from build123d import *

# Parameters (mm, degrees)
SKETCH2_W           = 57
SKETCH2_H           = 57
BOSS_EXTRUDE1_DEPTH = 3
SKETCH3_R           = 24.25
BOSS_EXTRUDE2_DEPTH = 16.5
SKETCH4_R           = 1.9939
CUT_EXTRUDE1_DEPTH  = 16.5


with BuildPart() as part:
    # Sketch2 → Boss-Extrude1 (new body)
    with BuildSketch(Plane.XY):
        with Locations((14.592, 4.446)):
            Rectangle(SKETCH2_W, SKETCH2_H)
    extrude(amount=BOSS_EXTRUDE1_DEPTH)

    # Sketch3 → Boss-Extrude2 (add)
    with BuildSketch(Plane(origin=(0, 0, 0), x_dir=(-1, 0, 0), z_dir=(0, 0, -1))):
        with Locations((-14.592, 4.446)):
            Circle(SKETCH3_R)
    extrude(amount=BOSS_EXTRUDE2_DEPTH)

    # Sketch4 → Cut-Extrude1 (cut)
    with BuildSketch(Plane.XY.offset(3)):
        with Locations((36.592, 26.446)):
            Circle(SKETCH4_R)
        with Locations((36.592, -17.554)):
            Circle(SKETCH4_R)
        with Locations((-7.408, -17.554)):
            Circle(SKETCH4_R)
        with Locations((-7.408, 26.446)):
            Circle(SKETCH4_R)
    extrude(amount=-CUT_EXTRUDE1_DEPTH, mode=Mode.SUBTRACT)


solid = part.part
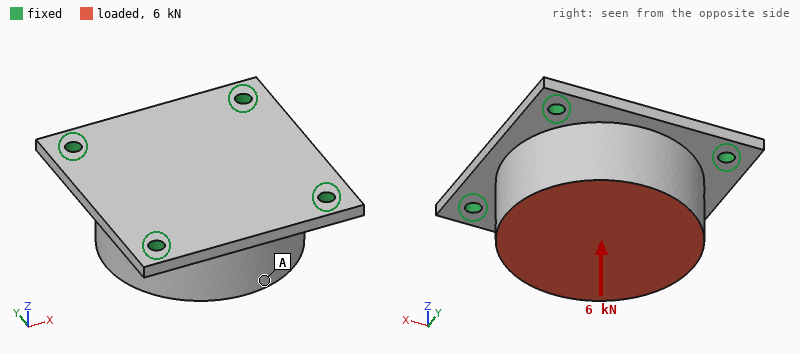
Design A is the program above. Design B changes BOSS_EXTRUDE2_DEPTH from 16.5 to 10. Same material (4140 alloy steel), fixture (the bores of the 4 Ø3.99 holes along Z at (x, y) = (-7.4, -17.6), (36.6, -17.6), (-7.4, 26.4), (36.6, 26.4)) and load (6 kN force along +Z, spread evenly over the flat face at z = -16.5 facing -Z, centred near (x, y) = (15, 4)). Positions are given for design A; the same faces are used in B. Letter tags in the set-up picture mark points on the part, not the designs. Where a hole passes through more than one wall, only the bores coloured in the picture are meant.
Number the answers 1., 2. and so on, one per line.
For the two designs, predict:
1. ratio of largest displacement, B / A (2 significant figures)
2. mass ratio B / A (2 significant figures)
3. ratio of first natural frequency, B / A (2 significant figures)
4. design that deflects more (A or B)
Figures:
1. 1.1
2. 0.70
3. 1.2
4. B
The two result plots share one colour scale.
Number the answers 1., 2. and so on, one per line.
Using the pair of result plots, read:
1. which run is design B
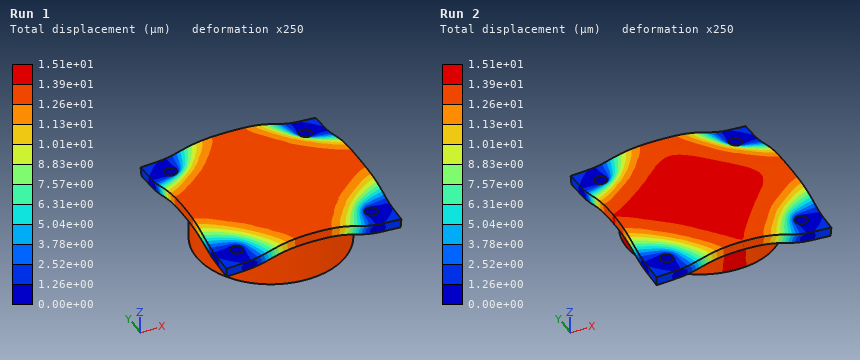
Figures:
1. Run 2
